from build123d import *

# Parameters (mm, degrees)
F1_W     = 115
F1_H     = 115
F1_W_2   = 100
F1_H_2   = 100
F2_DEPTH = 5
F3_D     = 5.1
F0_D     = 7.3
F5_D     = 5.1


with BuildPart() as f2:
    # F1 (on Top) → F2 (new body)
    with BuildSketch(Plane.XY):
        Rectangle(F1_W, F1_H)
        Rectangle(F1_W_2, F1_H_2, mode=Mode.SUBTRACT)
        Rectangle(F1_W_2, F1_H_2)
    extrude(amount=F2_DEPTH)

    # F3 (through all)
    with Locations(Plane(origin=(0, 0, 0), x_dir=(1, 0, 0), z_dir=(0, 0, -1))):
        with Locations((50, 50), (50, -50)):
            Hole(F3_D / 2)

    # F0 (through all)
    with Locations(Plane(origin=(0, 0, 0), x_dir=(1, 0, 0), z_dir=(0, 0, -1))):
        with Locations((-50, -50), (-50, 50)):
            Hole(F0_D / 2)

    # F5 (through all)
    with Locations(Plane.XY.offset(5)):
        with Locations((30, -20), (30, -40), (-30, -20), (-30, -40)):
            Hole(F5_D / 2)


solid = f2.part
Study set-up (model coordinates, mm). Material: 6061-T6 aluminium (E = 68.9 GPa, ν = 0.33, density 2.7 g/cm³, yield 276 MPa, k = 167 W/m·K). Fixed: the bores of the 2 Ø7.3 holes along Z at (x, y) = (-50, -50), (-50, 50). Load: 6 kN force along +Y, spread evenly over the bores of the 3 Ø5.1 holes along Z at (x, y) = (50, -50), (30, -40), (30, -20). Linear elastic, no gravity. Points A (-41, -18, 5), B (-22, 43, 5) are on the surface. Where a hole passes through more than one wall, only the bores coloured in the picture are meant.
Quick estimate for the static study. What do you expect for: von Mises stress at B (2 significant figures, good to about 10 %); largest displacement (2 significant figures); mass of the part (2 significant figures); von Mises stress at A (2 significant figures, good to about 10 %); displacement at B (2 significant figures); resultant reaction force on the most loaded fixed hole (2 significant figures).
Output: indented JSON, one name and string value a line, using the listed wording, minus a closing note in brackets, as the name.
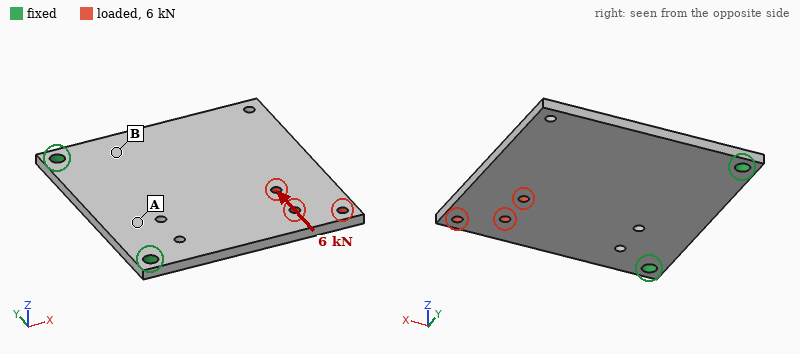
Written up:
{
  "von Mises stress at B": "31 MPa",
  "largest displacement": "0.11 mm",
  "mass of the part": "180 g",
  "von Mises stress at A": "12 MPa",
  "displacement at B": "0.025 mm",
  "resultant reaction force on the most loaded fixed hole": "6.0 kN"
}
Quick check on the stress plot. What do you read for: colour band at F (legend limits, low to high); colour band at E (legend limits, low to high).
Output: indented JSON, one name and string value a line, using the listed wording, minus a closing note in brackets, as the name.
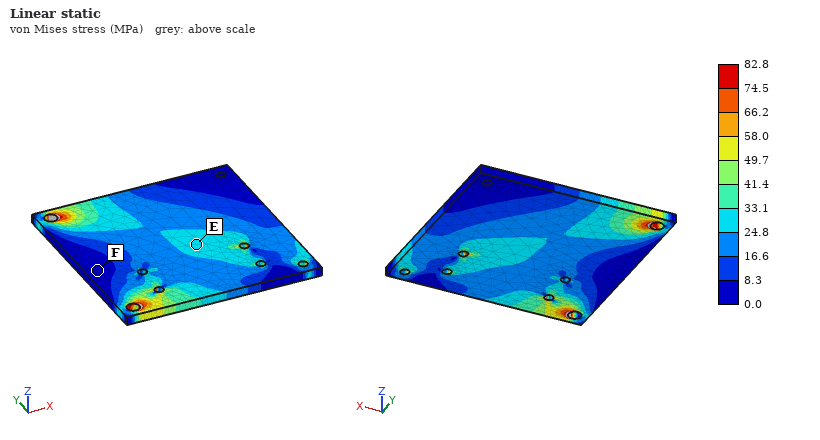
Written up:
{
  "colour band at F": "0.0 to 8.3 MPa",
  "colour band at E": "24.8 to 33.1 MPa"
}
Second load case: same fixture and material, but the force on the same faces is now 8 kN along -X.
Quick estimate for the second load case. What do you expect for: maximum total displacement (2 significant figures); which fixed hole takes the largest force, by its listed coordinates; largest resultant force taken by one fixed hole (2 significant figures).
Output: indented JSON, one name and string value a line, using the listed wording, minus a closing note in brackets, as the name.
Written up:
{
  "maximum total displacement": "85 µm",
  "which fixed hole takes the largest force, by its listed coordinates": "(-50, -50)",
  "largest resultant force taken by one fixed hole": "7.1 kN"
}
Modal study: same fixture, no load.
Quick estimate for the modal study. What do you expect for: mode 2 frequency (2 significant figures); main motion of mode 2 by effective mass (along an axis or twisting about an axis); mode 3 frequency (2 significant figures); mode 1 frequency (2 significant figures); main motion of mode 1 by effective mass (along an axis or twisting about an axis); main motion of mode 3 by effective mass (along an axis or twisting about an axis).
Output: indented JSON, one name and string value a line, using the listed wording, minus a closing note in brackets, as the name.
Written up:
{
  "mode 2 frequency": "840 Hz",
  "main motion of mode 2 by effective mass": "twisting about X",
  "mode 3 frequency": "1900 Hz",
  "mode 1 frequency": "290 Hz",
  "main motion of mode 1 by effective mass": "along Z",
  "main motion of mode 3 by effective mass": "along Z"
}
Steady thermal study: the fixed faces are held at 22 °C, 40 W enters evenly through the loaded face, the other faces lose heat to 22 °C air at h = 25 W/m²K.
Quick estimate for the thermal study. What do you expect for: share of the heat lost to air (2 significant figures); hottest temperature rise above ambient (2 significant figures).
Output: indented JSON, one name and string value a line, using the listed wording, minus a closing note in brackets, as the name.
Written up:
{
  "share of the heat lost to air": "36 %",
  "hottest temperature rise above ambient": "54 K"
}
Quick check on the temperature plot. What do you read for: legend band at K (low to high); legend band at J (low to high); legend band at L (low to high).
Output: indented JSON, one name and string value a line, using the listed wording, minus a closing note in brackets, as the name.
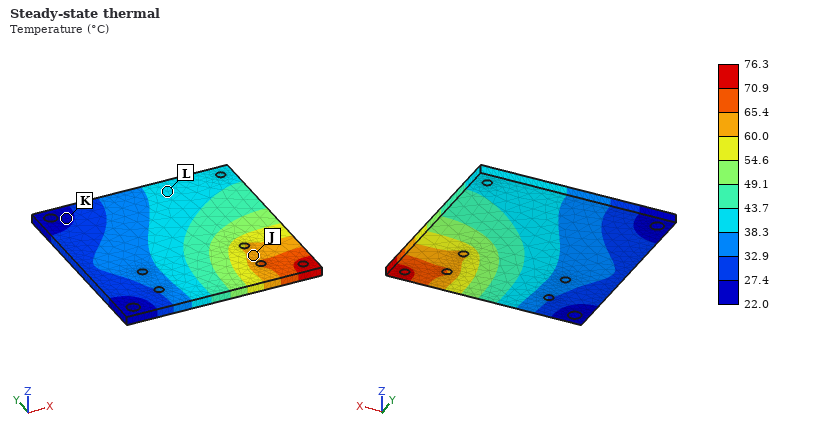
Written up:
{
  "legend band at K": "22.0 to 27.4 °C",
  "legend band at J": "60.0 to 65.4 °C",
  "legend band at L": "38.3 to 43.7 °C"
}
